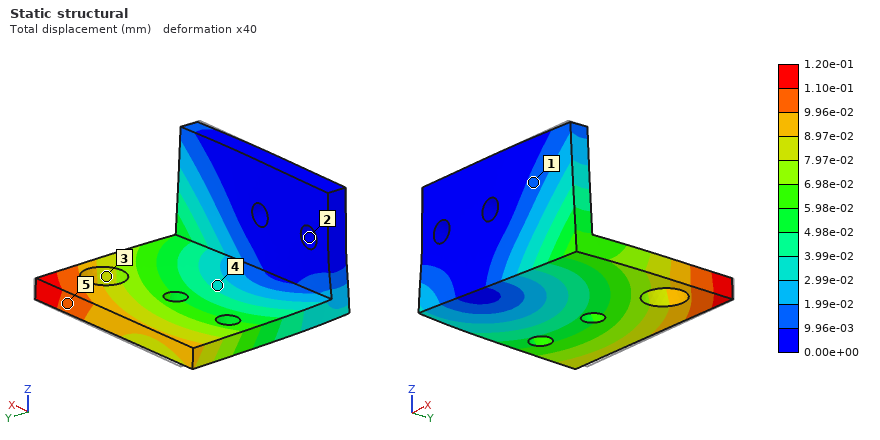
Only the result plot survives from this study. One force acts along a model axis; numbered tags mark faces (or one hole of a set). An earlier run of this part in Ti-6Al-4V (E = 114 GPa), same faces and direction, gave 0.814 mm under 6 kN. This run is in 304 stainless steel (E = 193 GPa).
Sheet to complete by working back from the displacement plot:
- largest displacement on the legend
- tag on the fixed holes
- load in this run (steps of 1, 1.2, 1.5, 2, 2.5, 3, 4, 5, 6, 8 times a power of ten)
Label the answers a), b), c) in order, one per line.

a) 1.20e-01 mm
b) 2
c) 1.5 kN
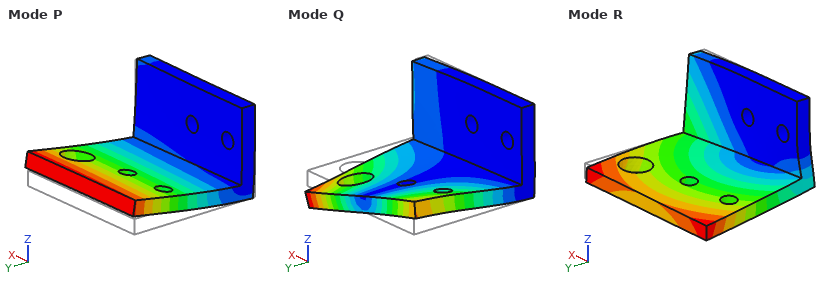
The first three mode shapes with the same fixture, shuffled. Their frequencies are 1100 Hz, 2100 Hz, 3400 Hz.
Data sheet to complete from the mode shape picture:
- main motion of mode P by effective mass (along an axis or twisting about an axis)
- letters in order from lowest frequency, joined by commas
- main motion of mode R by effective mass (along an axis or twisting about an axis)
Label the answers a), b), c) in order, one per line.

a) along Z
b) P, R, Q
c) along X
